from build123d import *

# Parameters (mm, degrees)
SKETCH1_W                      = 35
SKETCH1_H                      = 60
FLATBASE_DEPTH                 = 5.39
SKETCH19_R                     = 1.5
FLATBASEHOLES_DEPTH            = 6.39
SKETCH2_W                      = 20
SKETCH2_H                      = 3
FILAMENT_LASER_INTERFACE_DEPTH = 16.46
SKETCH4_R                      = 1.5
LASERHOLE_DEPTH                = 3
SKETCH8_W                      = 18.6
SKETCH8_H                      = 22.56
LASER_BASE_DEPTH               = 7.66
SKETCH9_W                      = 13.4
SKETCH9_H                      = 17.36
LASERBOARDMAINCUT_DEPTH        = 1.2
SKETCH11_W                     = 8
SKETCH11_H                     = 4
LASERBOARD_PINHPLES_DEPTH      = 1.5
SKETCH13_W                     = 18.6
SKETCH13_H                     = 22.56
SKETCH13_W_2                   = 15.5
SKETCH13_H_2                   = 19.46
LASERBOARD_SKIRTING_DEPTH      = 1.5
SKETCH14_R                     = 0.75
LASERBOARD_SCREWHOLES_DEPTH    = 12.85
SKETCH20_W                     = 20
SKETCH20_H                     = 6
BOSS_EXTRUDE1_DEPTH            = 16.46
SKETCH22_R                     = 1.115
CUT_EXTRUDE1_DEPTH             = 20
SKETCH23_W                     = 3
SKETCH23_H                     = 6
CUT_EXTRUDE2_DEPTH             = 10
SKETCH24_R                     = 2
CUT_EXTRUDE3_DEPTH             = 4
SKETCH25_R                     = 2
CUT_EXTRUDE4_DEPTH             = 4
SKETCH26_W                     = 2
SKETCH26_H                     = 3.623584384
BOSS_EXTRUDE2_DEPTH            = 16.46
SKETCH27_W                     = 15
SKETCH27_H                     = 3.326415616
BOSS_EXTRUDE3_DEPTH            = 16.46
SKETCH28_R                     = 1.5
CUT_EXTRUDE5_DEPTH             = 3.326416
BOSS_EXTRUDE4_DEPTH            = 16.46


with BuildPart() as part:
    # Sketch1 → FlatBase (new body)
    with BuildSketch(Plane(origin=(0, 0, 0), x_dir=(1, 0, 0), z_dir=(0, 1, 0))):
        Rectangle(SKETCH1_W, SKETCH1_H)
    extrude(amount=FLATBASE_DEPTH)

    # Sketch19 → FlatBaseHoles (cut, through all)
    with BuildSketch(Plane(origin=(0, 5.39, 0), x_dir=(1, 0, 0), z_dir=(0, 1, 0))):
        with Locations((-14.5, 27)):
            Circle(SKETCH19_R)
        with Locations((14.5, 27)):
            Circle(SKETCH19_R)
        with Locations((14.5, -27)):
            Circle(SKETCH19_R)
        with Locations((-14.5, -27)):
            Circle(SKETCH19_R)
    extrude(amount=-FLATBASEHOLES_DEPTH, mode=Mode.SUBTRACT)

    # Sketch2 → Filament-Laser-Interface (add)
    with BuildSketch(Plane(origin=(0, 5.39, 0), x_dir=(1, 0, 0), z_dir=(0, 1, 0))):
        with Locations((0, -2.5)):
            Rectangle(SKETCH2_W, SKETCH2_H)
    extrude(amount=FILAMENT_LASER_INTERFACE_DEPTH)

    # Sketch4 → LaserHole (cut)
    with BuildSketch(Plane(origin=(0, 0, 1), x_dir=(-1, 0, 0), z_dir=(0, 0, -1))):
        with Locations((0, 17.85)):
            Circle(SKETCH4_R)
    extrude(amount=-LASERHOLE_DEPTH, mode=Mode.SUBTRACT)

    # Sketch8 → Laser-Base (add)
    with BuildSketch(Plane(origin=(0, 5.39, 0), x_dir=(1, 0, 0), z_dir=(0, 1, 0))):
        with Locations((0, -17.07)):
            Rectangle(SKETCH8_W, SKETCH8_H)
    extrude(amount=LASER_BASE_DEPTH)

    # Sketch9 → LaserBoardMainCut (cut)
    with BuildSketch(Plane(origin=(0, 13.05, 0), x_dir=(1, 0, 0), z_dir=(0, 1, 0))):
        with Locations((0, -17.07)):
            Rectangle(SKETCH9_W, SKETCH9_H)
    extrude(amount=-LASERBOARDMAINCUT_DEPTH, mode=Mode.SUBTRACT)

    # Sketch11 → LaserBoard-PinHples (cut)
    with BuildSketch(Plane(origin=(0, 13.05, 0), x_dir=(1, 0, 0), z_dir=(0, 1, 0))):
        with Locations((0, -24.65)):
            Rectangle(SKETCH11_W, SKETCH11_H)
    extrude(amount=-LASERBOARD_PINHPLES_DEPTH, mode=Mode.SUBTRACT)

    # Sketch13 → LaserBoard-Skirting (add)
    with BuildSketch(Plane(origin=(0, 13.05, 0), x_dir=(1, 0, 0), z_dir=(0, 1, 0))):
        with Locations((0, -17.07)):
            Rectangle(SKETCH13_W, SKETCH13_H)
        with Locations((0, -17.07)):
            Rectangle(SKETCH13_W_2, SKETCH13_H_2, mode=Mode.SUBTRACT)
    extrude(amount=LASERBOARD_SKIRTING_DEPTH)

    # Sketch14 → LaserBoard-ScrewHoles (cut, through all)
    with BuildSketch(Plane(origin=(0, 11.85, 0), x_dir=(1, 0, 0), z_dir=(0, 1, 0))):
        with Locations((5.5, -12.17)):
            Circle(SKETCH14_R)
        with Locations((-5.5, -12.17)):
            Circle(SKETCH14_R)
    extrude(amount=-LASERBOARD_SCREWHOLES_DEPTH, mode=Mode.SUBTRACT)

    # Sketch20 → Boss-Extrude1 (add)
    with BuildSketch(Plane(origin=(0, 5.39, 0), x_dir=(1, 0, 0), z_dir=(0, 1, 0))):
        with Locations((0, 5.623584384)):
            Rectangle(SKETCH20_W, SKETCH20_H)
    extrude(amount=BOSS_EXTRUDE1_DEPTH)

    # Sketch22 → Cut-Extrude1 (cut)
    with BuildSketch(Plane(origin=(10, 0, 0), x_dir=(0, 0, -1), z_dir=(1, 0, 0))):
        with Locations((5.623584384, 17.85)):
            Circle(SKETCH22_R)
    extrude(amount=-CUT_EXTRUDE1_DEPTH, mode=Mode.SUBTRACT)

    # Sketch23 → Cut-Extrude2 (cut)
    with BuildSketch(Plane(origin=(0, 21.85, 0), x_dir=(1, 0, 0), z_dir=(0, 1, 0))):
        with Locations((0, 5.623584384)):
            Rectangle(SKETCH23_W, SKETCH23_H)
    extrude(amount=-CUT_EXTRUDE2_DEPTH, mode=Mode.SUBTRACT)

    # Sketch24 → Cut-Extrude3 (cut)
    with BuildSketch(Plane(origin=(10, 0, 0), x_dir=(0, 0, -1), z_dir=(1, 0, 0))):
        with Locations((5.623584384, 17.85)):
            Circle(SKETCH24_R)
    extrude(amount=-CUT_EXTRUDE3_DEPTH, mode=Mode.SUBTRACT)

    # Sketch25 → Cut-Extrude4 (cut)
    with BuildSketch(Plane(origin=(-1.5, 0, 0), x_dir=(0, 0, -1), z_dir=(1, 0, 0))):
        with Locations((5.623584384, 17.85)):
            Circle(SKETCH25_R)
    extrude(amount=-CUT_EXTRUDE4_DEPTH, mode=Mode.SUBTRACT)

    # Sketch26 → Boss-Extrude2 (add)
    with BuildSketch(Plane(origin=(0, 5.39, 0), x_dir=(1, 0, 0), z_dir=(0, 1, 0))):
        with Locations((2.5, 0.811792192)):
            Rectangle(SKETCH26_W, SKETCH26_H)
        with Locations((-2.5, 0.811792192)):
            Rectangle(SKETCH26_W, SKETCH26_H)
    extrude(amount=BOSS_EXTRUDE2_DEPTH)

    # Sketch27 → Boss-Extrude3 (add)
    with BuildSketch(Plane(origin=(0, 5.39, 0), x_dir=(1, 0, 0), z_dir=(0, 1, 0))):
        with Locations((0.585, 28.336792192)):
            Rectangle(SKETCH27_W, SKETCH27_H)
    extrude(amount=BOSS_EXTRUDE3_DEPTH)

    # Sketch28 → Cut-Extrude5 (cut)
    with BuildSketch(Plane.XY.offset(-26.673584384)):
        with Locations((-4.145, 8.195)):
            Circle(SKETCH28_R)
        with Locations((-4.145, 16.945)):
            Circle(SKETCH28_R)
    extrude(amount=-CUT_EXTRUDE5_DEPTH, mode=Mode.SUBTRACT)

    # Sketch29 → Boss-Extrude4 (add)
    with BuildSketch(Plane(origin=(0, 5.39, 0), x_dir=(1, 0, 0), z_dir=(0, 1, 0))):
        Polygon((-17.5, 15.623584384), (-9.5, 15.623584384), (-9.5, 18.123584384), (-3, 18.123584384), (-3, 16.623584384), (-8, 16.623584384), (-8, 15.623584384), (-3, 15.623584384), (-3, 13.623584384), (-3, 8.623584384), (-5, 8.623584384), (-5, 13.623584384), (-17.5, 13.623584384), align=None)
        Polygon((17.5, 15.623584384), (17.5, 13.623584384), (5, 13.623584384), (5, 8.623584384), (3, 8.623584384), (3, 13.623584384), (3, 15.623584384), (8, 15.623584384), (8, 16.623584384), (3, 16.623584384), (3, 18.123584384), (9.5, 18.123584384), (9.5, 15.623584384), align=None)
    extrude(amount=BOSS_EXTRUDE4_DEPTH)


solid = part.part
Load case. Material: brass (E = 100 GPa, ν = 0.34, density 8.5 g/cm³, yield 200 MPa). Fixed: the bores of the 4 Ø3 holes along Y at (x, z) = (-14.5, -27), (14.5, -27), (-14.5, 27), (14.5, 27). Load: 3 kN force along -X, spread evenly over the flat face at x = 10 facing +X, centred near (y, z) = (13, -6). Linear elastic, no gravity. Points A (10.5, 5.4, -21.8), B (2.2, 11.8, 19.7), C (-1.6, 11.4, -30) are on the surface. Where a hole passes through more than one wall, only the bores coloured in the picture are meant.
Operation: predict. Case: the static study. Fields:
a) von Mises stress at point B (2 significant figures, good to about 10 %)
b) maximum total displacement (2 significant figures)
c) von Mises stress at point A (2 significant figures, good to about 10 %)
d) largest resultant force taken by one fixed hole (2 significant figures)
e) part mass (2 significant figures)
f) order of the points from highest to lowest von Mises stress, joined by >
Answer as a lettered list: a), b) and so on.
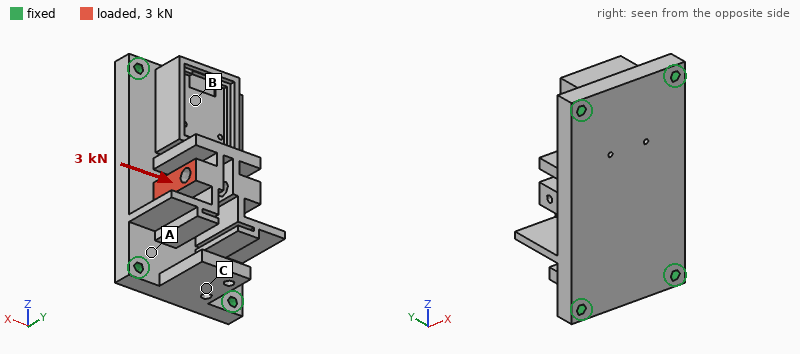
a) 24 MPa
b) 64 µm
c) 51 MPa
d) 1.2 kN
e) 170 g
f) A > B > C
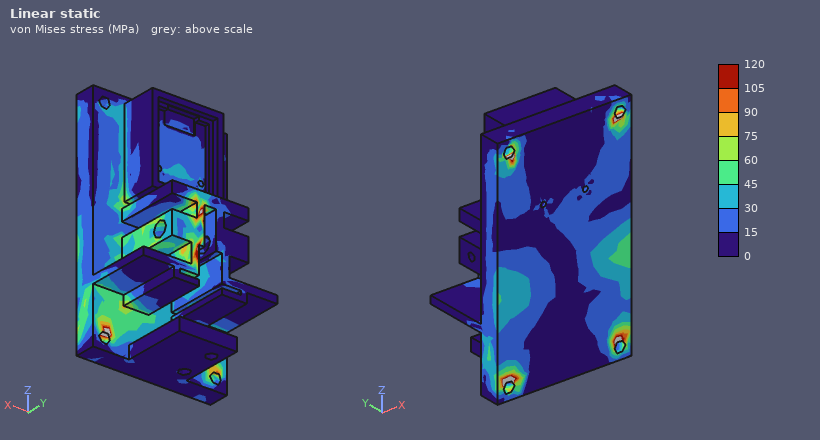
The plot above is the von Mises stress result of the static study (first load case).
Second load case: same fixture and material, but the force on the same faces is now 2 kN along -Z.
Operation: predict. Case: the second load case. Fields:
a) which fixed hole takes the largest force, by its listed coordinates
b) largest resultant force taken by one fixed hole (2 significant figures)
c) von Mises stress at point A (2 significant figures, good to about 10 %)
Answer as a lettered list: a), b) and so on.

a) (14.5, -27)
b) 720 N
c) 19 MPa
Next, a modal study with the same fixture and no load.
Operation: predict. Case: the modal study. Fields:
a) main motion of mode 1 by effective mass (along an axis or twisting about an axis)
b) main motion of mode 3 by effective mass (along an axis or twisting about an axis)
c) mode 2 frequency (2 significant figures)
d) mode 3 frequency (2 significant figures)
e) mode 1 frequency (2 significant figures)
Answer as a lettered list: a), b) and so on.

a) along Y
b) along X
c) 5200 Hz
d) 6800 Hz
e) 4200 Hz
